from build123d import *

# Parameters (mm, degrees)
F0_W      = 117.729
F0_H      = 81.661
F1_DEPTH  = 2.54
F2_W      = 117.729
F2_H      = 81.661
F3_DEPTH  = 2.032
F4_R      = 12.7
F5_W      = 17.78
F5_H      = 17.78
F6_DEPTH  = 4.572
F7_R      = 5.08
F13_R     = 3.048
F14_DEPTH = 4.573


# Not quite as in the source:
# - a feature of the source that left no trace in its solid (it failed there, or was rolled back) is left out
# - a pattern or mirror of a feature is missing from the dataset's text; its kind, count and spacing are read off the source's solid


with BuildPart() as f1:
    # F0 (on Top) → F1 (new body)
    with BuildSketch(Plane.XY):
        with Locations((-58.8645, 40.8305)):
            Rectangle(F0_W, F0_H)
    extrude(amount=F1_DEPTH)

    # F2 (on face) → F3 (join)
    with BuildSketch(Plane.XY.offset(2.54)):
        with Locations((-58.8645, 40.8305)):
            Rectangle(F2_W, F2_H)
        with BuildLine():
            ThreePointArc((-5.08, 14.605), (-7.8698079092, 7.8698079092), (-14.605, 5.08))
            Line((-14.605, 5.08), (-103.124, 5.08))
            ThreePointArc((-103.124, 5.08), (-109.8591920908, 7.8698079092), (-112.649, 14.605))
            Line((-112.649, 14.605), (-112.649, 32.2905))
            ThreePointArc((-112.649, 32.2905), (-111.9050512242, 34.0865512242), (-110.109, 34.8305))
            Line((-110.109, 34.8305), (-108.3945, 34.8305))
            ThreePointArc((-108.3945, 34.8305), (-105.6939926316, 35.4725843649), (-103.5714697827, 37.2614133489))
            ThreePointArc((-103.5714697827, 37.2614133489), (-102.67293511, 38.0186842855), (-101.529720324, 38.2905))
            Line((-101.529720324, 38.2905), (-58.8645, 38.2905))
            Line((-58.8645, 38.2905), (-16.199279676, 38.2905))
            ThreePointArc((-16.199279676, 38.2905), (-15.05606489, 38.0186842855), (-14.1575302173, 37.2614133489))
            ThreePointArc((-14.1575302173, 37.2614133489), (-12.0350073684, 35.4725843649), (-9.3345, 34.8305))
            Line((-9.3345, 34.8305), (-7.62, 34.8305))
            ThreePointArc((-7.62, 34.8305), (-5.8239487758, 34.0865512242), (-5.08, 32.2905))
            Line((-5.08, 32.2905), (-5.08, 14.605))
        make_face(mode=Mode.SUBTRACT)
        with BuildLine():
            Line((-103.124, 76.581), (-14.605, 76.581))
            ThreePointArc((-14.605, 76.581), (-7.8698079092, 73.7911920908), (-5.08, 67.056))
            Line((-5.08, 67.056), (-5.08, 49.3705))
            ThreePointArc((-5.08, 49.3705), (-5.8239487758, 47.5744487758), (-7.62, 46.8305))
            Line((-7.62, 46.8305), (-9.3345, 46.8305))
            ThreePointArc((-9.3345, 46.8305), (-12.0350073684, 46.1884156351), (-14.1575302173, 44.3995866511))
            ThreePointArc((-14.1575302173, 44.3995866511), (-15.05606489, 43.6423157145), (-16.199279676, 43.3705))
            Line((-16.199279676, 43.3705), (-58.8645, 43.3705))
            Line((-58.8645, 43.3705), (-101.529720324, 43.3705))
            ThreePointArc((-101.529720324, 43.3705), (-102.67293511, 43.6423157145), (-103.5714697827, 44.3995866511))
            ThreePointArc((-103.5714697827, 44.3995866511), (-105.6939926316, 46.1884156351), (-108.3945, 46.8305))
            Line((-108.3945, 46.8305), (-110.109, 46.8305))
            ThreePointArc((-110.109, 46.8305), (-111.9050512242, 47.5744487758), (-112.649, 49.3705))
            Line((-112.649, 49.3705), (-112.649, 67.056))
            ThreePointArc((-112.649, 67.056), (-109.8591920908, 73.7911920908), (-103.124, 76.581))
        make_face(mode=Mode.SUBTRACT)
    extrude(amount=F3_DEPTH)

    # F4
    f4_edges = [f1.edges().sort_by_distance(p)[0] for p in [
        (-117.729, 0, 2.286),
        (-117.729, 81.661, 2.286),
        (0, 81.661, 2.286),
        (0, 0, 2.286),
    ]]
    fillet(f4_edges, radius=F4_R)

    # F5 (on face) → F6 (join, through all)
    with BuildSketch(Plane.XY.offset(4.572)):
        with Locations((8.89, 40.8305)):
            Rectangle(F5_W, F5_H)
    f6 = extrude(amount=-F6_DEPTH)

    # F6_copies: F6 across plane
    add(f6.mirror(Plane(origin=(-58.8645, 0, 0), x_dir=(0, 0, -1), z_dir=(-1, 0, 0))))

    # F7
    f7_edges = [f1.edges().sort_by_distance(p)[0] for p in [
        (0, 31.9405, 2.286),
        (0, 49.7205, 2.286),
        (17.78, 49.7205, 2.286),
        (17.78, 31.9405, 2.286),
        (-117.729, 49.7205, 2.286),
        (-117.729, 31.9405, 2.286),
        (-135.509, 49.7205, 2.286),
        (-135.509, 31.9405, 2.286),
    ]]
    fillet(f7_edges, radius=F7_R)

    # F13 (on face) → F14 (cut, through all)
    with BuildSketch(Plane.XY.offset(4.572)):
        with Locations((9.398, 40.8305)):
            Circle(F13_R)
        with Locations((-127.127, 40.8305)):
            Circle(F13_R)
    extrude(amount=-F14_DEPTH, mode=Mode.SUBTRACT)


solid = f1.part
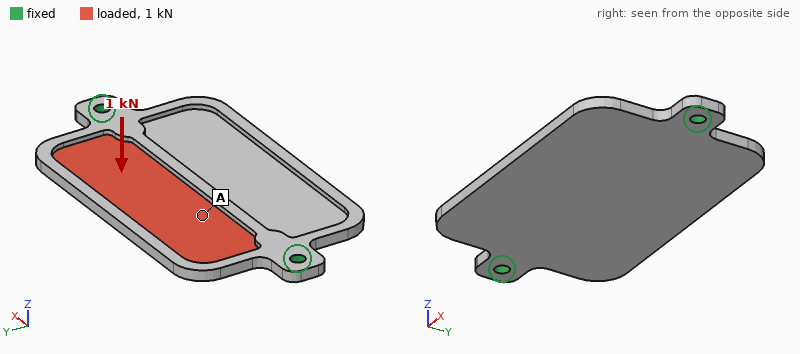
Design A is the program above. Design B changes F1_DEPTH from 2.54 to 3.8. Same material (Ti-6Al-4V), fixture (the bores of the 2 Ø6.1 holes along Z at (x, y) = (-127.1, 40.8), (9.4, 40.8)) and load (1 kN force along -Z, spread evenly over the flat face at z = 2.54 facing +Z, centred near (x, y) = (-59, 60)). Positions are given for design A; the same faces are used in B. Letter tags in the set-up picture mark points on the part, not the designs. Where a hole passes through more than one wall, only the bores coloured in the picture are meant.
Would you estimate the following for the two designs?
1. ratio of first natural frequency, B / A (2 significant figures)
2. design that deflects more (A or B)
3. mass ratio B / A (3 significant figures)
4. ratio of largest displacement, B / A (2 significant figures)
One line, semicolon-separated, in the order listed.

1.0; A; 1.28; 0.75
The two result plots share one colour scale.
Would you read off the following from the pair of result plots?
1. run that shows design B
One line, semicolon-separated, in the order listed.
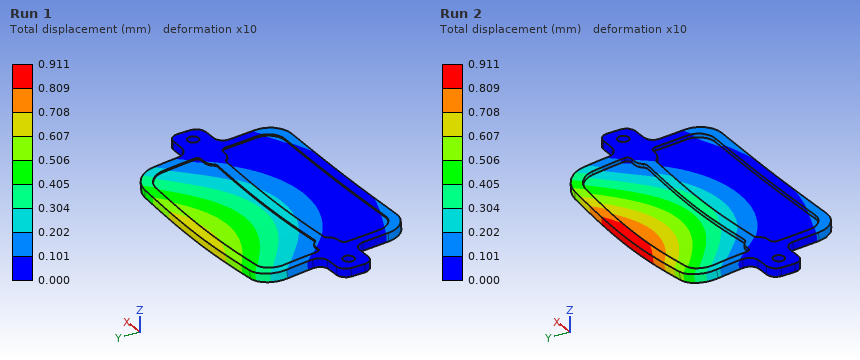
Run 1
